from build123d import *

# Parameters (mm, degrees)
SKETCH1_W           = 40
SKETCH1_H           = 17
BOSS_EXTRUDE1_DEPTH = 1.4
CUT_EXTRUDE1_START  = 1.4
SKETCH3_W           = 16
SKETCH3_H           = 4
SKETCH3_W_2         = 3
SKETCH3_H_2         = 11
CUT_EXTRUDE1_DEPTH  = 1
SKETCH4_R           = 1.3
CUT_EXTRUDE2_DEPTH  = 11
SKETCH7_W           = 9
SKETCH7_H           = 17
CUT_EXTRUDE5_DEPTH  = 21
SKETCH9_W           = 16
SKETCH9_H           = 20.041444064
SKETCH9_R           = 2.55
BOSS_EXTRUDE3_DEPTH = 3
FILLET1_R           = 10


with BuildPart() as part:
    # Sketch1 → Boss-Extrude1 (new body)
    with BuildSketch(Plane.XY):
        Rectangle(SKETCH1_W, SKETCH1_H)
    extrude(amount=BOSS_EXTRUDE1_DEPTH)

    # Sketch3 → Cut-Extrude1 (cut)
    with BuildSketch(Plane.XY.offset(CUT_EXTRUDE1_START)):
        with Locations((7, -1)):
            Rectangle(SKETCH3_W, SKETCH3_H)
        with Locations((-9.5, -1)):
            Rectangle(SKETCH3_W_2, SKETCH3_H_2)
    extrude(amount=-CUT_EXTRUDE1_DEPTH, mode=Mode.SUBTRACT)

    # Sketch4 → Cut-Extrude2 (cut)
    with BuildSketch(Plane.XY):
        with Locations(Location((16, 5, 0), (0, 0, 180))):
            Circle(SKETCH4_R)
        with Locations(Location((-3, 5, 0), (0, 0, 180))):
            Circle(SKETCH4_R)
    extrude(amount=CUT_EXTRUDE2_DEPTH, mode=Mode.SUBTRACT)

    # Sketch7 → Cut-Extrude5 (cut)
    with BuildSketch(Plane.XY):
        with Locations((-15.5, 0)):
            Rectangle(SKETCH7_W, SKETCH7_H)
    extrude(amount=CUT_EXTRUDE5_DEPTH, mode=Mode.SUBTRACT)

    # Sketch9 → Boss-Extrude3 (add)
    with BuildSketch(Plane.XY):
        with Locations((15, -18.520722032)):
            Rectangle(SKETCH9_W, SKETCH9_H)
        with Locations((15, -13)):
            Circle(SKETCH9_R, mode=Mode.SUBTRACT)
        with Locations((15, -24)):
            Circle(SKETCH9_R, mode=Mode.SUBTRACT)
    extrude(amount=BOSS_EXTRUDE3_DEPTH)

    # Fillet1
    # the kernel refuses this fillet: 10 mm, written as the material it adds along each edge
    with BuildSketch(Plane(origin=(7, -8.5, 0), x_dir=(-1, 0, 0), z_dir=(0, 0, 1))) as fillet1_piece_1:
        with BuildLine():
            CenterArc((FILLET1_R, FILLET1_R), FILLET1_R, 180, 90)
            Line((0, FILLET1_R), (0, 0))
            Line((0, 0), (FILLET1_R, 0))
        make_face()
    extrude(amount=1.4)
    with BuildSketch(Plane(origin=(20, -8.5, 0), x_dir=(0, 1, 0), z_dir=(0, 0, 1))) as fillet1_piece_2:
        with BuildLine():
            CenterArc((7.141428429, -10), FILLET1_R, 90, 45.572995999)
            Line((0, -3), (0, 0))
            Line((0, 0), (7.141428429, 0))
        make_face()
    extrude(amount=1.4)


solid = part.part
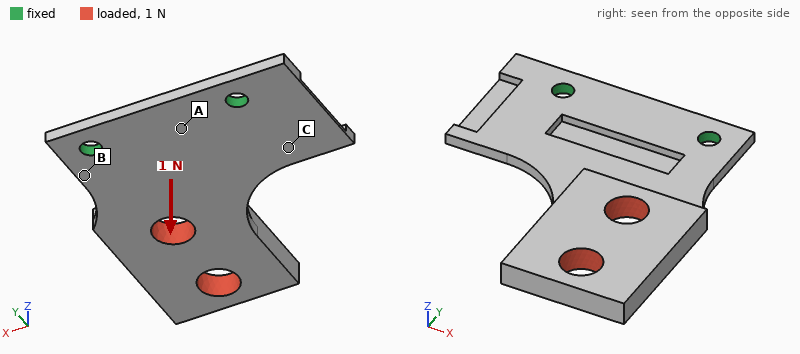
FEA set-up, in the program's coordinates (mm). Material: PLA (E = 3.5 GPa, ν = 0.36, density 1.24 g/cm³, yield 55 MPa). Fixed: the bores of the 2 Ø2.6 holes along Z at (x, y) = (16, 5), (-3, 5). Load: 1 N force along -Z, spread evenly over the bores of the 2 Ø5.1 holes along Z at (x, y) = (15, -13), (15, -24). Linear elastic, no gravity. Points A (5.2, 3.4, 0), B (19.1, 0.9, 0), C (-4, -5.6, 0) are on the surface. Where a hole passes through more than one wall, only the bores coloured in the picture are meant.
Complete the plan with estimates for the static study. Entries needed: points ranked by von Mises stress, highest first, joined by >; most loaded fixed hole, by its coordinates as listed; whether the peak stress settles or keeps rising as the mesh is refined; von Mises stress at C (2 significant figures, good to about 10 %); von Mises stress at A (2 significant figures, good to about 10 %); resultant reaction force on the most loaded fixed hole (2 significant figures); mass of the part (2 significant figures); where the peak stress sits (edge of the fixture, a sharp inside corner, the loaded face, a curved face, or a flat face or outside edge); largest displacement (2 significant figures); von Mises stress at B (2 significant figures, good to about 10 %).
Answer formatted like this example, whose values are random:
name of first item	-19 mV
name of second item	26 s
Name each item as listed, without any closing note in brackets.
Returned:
points ranked by von Mises stress, highest first, joined by >	B > C > A
most loaded fixed hole, by its coordinates as listed	(16, 5)
whether the peak stress settles or keeps rising as the mesh is refined	keeps rising
von Mises stress at C	1.8 MPa
von Mises stress at A	0.62 MPa
resultant reaction force on the most loaded fixed hole	1.1 N
mass of the part	1.9 g
where the peak stress sits	a sharp inside corner
largest displacement	0.54 mm
von Mises stress at B	4.7 MPa
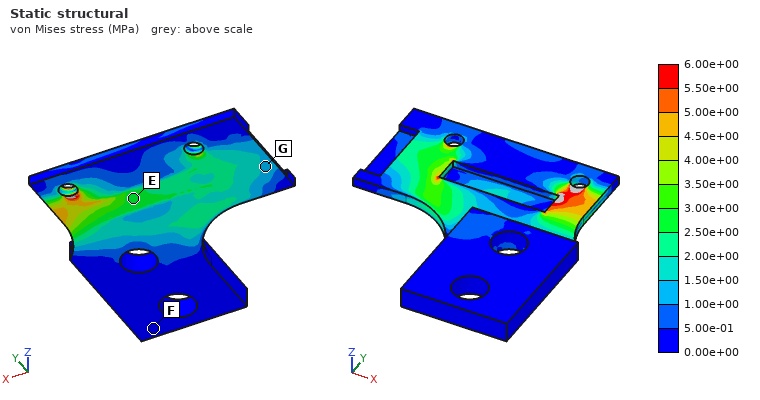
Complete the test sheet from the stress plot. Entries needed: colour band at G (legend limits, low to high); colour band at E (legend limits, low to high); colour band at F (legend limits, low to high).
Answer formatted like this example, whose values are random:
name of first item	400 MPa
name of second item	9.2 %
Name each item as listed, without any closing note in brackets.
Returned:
colour band at G	1.00e+00 to 1.50e+00 MPa
colour band at E	2.50e+00 to 3.00e+00 MPa
colour band at F	0.00e+00 to 5.00e-01 MPa
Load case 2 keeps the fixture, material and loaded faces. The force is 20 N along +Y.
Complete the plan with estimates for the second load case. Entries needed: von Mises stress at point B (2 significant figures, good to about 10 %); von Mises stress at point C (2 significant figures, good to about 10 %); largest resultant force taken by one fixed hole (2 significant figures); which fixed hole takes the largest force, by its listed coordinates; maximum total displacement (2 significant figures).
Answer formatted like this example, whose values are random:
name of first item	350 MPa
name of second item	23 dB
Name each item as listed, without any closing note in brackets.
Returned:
von Mises stress at point B	2.4 MPa
von Mises stress at point C	2.0 MPa
largest resultant force taken by one fixed hole	18 N
which fixed hole takes the largest force, by its listed coordinates	(16, 5)
maximum total displacement	0.55 mm
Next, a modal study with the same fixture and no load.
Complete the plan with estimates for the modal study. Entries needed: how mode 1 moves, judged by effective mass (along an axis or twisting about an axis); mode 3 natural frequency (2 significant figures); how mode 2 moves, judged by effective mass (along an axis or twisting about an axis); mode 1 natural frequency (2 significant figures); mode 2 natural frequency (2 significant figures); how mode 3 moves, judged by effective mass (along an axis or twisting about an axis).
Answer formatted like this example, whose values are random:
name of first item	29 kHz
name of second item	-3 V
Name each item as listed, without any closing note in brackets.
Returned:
how mode 1 moves, judged by effective mass	along Z
mode 3 natural frequency	2300 Hz
how mode 2 moves, judged by effective mass	twisting about Y
mode 1 natural frequency	260 Hz
mode 2 natural frequency	1400 Hz
how mode 3 moves, judged by effective mass	along Z
